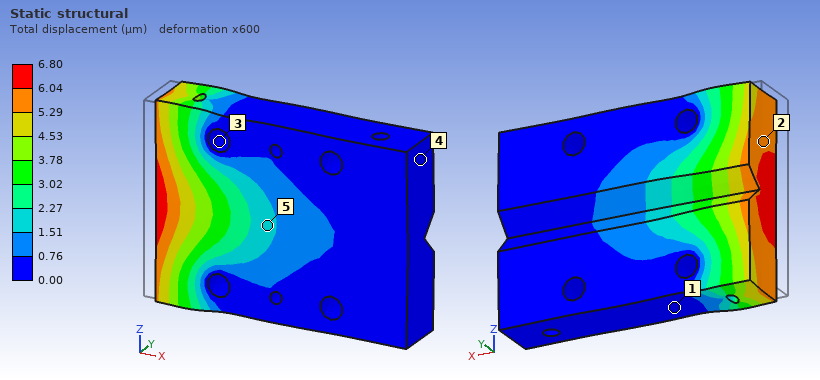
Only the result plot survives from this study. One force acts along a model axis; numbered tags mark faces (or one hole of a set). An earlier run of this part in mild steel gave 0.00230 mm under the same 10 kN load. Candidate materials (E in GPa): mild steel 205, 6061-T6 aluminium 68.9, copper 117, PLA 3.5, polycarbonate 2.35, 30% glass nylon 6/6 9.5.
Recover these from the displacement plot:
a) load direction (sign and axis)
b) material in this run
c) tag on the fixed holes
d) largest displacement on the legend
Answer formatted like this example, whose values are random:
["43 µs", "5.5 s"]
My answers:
["+X", "6061-T6 aluminium", "3", "6.80 µm"]
